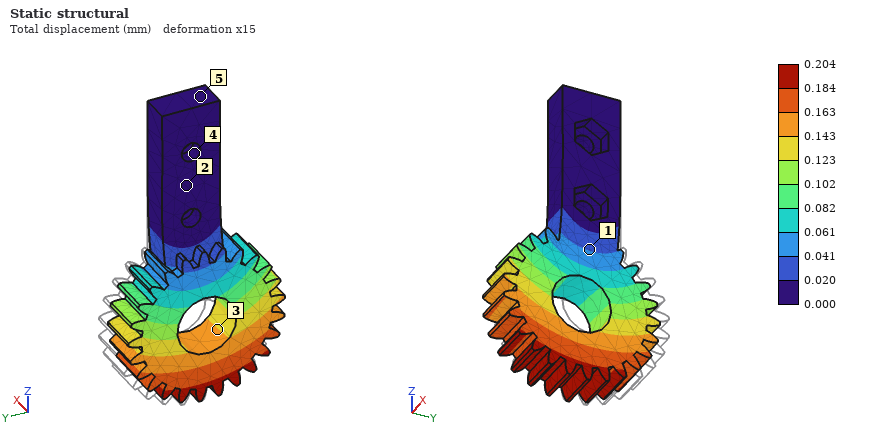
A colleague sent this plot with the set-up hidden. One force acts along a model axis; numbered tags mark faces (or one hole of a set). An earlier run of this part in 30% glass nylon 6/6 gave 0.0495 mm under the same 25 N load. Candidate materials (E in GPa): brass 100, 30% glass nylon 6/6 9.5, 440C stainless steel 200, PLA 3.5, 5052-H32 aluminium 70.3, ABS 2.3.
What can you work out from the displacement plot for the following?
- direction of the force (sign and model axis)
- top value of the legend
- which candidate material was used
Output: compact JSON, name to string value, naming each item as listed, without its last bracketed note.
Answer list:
{"direction of the force": "-Y", "top value of the legend": "0.204 mm", "which candidate material was used": "ABS"}
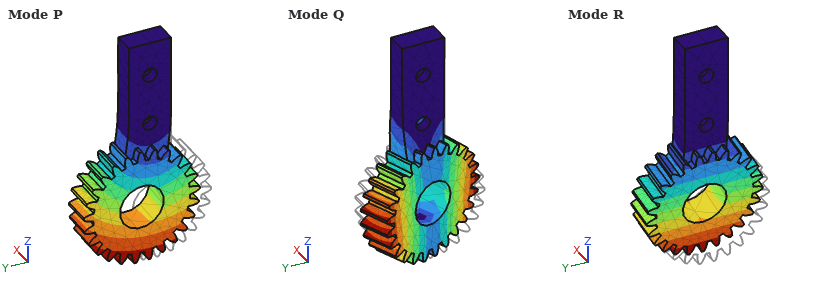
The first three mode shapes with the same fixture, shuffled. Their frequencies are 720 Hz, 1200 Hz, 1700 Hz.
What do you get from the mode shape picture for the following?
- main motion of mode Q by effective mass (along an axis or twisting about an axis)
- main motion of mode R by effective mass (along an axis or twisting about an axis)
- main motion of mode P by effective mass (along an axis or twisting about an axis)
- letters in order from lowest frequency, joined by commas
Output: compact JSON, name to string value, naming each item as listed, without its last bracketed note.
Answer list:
{"main motion of mode Q by effective mass": "twisting about Z", "main motion of mode R by effective mass": "along X", "main motion of mode P by effective mass": "along Y", "letters in order from lowest frequency, joined by commas": "R, P, Q"}
